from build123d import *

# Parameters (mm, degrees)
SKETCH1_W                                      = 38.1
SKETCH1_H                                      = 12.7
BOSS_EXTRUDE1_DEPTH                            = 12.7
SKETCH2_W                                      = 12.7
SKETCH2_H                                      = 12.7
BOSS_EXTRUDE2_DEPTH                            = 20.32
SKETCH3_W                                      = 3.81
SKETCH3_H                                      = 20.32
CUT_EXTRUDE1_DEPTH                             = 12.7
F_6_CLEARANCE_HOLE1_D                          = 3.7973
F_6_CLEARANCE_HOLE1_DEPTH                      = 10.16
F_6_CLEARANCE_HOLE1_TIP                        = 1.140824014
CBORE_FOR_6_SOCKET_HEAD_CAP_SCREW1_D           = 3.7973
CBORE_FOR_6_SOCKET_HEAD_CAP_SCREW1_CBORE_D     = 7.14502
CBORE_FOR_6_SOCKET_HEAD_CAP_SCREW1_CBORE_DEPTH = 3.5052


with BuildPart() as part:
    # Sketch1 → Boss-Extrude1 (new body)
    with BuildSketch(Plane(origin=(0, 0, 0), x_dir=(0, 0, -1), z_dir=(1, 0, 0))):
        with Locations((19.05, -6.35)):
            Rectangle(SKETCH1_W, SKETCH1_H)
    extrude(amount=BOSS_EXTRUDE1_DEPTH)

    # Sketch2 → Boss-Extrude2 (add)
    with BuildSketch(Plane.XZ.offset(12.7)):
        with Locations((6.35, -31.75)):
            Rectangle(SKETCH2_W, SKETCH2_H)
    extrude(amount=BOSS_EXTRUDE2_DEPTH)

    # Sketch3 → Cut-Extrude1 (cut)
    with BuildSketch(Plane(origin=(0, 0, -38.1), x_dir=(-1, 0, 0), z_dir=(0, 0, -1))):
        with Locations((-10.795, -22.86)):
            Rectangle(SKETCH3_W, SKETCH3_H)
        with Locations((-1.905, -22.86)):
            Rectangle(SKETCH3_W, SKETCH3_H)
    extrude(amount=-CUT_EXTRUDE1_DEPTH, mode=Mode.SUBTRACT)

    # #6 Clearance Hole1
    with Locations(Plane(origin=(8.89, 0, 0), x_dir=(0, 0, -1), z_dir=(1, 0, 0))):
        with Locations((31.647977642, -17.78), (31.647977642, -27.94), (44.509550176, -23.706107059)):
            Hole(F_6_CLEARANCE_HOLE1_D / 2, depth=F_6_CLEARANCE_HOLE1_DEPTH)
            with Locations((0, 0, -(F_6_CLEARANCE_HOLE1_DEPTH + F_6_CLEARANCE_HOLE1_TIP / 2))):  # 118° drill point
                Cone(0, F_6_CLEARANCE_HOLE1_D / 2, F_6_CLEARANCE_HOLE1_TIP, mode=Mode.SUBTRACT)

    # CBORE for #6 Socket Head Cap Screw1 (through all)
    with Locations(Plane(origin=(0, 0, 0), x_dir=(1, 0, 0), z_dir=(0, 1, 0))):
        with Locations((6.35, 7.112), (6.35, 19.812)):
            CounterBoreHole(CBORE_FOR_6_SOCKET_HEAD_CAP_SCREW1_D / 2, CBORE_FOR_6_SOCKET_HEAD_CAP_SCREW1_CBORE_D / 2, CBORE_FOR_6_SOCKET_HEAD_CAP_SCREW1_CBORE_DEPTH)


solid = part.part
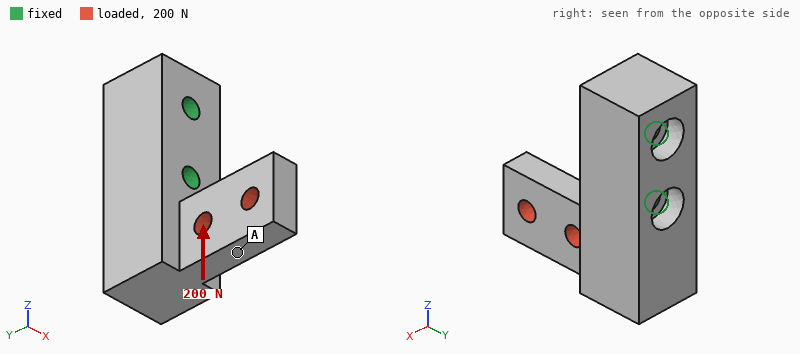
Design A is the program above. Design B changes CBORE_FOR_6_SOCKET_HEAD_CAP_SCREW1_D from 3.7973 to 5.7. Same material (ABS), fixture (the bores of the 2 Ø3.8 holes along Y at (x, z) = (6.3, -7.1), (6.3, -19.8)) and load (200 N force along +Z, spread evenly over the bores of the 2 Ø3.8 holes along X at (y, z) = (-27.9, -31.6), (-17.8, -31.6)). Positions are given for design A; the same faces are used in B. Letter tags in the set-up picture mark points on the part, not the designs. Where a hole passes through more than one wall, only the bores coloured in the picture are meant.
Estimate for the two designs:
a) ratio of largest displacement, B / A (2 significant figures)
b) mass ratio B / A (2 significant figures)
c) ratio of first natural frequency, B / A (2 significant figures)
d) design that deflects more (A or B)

0.92
0.96
1.0
A
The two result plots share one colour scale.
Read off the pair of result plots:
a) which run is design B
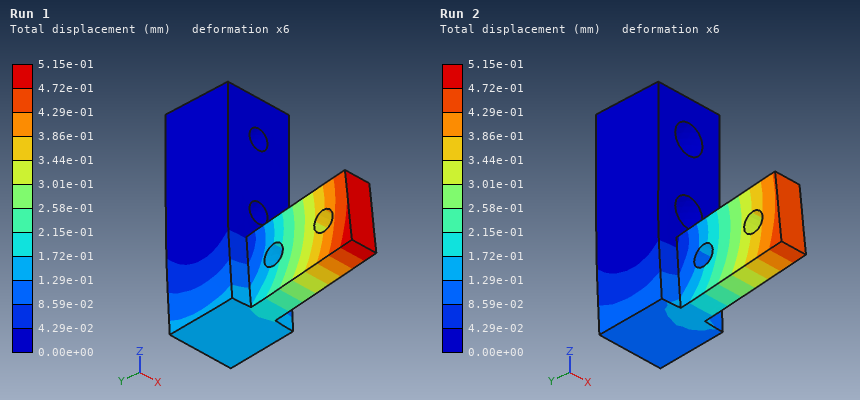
Run 2
